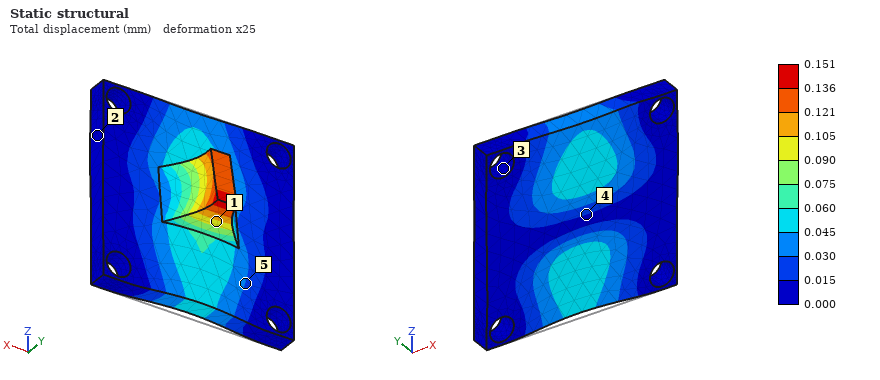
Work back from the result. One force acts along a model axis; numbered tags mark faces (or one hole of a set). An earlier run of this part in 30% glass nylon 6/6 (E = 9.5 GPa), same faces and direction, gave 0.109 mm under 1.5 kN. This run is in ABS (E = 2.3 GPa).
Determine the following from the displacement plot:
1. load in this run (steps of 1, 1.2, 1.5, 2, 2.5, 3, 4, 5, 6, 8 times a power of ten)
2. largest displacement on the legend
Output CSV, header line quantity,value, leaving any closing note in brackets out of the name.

quantity,value
load in this run,500 N
largest displacement on the legend,0.151 mm
